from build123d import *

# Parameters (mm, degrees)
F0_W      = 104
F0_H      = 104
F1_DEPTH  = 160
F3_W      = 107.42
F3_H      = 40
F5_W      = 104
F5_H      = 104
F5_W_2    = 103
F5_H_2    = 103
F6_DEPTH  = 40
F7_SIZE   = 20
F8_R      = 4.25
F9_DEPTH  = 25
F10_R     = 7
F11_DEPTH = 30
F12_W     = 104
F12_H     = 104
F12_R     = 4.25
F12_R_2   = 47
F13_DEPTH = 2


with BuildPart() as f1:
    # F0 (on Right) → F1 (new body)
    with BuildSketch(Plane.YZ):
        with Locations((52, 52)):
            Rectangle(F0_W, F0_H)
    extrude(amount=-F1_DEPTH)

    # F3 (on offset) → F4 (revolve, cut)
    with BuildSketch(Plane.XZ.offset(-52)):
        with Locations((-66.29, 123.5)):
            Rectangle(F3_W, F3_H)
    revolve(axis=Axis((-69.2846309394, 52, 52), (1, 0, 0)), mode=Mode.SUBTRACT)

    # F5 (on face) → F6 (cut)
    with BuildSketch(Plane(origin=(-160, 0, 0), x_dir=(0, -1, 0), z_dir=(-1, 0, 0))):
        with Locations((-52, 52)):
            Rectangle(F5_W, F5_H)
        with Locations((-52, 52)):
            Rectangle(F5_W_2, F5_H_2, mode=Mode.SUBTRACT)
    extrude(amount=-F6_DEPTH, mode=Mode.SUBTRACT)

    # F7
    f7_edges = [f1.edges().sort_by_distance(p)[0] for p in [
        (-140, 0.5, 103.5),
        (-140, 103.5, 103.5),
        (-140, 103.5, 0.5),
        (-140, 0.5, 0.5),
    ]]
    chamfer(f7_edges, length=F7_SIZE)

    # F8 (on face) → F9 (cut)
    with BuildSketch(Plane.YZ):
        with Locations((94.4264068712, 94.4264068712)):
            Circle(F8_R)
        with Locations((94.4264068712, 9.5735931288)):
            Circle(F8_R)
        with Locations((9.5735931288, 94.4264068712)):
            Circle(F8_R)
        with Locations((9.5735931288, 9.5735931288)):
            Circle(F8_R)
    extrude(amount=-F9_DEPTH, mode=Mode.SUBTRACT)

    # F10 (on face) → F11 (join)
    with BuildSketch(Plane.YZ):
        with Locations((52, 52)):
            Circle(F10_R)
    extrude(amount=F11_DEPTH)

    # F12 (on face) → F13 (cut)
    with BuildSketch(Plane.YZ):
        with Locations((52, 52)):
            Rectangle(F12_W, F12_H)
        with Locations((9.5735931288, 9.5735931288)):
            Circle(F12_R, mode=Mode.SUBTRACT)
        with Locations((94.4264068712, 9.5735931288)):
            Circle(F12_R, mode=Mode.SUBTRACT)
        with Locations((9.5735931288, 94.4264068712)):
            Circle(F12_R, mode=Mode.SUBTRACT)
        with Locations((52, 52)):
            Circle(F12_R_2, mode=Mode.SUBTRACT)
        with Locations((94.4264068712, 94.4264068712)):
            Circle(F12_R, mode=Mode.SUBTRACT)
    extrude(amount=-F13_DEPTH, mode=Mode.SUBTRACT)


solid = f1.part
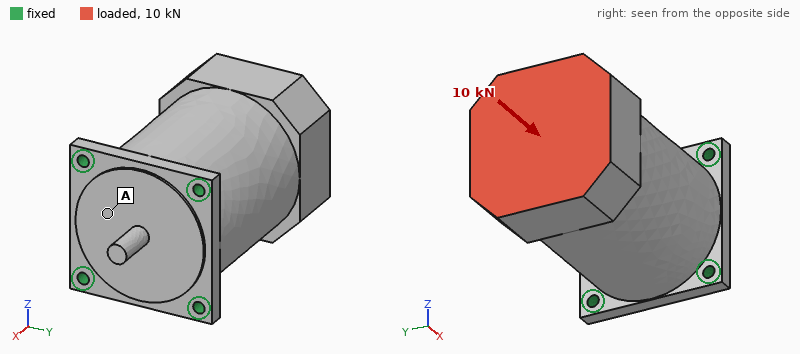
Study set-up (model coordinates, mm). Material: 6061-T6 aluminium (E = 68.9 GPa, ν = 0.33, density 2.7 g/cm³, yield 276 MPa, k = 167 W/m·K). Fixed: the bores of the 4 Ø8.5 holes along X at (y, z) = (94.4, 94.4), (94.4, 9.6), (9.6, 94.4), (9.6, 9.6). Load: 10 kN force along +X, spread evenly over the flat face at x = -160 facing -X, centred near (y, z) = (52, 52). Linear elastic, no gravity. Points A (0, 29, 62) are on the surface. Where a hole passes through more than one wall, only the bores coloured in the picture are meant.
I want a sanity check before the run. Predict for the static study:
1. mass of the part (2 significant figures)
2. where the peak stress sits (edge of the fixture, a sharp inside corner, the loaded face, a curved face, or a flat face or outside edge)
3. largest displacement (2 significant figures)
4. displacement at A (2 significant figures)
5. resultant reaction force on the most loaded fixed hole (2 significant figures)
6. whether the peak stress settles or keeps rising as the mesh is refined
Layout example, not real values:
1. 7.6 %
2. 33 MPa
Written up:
1. 3.8 kg
2. edge of the fixture
3. 9.8 µm
4. 7.7 µm
5. 2.7 kN
6. keeps rising
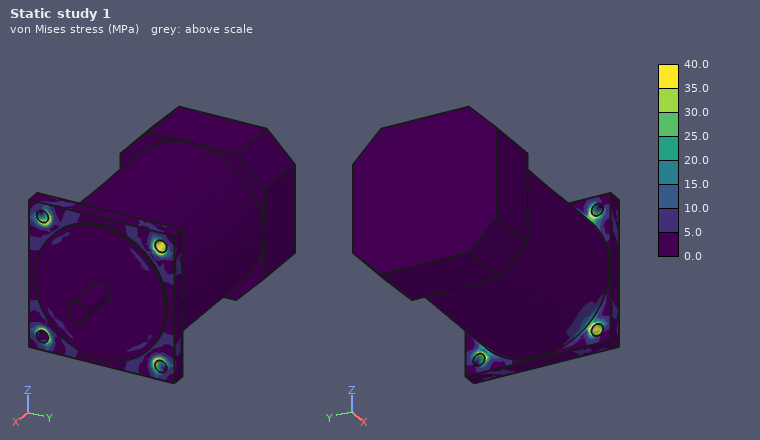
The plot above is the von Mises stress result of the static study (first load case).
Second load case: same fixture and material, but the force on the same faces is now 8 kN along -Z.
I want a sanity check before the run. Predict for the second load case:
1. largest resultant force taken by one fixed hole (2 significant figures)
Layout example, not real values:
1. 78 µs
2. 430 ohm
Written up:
1. 8.3 kN
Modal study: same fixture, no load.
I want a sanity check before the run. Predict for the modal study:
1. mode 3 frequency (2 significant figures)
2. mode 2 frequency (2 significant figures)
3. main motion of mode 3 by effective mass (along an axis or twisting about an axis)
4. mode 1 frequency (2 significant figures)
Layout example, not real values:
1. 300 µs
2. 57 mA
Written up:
1. 2900 Hz
2. 1200 Hz
3. along X
4. 1200 Hz
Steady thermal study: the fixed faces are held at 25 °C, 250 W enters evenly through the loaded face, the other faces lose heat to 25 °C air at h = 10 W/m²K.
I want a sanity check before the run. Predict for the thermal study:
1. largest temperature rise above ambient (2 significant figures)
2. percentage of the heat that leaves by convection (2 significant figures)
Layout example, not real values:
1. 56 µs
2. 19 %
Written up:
1. 41 K
2. 7.0 %
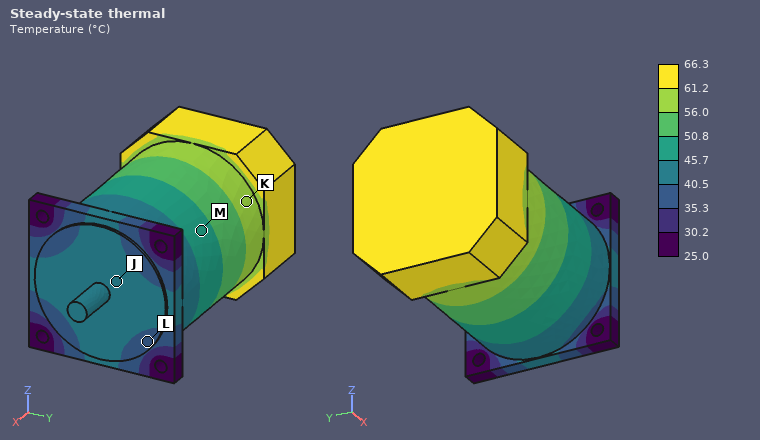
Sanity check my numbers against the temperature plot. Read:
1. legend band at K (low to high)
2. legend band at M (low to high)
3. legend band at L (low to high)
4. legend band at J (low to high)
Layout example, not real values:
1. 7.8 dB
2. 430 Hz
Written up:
1. 56.0 to 61.2 °C
2. 45.7 to 50.8 °C
3. 35.3 to 40.5 °C
4. 40.5 to 45.7 °C
